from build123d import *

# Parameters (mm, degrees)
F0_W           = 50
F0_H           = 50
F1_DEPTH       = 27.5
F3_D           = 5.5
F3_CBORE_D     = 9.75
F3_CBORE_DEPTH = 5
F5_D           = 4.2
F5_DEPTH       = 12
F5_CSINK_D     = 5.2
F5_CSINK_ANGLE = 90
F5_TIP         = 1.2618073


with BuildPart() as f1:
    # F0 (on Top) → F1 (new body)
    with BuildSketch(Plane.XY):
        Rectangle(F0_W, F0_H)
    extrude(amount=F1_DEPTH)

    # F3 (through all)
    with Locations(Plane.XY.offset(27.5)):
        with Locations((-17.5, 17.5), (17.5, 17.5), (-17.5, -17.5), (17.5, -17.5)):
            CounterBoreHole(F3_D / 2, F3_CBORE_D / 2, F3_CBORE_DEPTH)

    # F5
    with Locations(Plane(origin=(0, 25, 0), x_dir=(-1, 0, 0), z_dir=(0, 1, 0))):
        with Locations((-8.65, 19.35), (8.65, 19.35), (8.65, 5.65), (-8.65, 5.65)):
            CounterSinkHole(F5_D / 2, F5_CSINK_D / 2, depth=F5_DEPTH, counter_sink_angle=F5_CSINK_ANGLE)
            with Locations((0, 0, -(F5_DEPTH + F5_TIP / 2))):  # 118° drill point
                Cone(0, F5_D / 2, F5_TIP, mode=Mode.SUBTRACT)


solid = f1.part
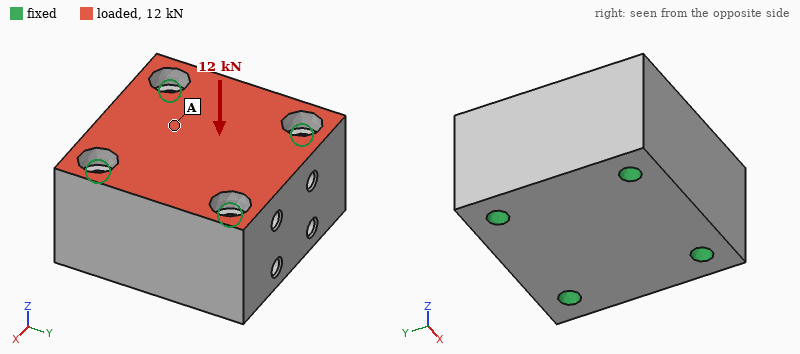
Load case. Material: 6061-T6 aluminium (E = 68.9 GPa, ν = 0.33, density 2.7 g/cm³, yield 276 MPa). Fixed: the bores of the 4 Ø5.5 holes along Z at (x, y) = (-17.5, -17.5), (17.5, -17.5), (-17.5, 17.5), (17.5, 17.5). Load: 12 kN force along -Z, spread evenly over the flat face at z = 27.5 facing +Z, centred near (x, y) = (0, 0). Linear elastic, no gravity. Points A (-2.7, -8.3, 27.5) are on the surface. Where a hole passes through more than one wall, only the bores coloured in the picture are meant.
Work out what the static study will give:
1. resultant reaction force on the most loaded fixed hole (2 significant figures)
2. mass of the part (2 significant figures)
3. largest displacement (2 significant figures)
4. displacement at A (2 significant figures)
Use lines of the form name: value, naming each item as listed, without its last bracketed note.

resultant reaction force on the most loaded fixed hole: 3.1 kN
mass of the part: 170 g
largest displacement: 3.2 µm
displacement at A: 3.0 µm
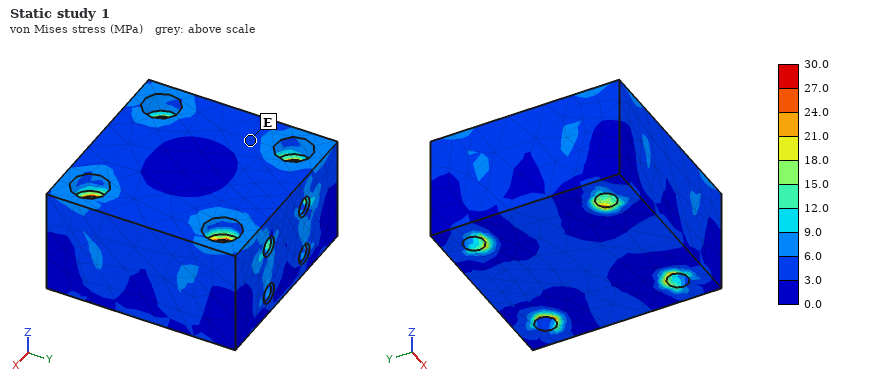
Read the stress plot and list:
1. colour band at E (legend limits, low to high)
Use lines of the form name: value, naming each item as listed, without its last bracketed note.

colour band at E: 3.0 to 6.0 MPa
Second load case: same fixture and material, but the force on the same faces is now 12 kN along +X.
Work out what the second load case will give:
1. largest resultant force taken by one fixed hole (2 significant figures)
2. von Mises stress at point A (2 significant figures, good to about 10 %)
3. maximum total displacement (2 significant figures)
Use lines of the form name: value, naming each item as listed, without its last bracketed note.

largest resultant force taken by one fixed hole: 3.6 kN
von Mises stress at point A: 11 MPa
maximum total displacement: 7.4 µm
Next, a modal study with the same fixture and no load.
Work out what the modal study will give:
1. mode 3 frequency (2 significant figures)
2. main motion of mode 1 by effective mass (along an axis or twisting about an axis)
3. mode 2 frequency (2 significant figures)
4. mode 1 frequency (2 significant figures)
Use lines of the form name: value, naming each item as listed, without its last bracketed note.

mode 3 frequency: 36 kHz
main motion of mode 1 by effective mass: along Z
mode 2 frequency: 35 kHz
mode 1 frequency: 30 kHz
